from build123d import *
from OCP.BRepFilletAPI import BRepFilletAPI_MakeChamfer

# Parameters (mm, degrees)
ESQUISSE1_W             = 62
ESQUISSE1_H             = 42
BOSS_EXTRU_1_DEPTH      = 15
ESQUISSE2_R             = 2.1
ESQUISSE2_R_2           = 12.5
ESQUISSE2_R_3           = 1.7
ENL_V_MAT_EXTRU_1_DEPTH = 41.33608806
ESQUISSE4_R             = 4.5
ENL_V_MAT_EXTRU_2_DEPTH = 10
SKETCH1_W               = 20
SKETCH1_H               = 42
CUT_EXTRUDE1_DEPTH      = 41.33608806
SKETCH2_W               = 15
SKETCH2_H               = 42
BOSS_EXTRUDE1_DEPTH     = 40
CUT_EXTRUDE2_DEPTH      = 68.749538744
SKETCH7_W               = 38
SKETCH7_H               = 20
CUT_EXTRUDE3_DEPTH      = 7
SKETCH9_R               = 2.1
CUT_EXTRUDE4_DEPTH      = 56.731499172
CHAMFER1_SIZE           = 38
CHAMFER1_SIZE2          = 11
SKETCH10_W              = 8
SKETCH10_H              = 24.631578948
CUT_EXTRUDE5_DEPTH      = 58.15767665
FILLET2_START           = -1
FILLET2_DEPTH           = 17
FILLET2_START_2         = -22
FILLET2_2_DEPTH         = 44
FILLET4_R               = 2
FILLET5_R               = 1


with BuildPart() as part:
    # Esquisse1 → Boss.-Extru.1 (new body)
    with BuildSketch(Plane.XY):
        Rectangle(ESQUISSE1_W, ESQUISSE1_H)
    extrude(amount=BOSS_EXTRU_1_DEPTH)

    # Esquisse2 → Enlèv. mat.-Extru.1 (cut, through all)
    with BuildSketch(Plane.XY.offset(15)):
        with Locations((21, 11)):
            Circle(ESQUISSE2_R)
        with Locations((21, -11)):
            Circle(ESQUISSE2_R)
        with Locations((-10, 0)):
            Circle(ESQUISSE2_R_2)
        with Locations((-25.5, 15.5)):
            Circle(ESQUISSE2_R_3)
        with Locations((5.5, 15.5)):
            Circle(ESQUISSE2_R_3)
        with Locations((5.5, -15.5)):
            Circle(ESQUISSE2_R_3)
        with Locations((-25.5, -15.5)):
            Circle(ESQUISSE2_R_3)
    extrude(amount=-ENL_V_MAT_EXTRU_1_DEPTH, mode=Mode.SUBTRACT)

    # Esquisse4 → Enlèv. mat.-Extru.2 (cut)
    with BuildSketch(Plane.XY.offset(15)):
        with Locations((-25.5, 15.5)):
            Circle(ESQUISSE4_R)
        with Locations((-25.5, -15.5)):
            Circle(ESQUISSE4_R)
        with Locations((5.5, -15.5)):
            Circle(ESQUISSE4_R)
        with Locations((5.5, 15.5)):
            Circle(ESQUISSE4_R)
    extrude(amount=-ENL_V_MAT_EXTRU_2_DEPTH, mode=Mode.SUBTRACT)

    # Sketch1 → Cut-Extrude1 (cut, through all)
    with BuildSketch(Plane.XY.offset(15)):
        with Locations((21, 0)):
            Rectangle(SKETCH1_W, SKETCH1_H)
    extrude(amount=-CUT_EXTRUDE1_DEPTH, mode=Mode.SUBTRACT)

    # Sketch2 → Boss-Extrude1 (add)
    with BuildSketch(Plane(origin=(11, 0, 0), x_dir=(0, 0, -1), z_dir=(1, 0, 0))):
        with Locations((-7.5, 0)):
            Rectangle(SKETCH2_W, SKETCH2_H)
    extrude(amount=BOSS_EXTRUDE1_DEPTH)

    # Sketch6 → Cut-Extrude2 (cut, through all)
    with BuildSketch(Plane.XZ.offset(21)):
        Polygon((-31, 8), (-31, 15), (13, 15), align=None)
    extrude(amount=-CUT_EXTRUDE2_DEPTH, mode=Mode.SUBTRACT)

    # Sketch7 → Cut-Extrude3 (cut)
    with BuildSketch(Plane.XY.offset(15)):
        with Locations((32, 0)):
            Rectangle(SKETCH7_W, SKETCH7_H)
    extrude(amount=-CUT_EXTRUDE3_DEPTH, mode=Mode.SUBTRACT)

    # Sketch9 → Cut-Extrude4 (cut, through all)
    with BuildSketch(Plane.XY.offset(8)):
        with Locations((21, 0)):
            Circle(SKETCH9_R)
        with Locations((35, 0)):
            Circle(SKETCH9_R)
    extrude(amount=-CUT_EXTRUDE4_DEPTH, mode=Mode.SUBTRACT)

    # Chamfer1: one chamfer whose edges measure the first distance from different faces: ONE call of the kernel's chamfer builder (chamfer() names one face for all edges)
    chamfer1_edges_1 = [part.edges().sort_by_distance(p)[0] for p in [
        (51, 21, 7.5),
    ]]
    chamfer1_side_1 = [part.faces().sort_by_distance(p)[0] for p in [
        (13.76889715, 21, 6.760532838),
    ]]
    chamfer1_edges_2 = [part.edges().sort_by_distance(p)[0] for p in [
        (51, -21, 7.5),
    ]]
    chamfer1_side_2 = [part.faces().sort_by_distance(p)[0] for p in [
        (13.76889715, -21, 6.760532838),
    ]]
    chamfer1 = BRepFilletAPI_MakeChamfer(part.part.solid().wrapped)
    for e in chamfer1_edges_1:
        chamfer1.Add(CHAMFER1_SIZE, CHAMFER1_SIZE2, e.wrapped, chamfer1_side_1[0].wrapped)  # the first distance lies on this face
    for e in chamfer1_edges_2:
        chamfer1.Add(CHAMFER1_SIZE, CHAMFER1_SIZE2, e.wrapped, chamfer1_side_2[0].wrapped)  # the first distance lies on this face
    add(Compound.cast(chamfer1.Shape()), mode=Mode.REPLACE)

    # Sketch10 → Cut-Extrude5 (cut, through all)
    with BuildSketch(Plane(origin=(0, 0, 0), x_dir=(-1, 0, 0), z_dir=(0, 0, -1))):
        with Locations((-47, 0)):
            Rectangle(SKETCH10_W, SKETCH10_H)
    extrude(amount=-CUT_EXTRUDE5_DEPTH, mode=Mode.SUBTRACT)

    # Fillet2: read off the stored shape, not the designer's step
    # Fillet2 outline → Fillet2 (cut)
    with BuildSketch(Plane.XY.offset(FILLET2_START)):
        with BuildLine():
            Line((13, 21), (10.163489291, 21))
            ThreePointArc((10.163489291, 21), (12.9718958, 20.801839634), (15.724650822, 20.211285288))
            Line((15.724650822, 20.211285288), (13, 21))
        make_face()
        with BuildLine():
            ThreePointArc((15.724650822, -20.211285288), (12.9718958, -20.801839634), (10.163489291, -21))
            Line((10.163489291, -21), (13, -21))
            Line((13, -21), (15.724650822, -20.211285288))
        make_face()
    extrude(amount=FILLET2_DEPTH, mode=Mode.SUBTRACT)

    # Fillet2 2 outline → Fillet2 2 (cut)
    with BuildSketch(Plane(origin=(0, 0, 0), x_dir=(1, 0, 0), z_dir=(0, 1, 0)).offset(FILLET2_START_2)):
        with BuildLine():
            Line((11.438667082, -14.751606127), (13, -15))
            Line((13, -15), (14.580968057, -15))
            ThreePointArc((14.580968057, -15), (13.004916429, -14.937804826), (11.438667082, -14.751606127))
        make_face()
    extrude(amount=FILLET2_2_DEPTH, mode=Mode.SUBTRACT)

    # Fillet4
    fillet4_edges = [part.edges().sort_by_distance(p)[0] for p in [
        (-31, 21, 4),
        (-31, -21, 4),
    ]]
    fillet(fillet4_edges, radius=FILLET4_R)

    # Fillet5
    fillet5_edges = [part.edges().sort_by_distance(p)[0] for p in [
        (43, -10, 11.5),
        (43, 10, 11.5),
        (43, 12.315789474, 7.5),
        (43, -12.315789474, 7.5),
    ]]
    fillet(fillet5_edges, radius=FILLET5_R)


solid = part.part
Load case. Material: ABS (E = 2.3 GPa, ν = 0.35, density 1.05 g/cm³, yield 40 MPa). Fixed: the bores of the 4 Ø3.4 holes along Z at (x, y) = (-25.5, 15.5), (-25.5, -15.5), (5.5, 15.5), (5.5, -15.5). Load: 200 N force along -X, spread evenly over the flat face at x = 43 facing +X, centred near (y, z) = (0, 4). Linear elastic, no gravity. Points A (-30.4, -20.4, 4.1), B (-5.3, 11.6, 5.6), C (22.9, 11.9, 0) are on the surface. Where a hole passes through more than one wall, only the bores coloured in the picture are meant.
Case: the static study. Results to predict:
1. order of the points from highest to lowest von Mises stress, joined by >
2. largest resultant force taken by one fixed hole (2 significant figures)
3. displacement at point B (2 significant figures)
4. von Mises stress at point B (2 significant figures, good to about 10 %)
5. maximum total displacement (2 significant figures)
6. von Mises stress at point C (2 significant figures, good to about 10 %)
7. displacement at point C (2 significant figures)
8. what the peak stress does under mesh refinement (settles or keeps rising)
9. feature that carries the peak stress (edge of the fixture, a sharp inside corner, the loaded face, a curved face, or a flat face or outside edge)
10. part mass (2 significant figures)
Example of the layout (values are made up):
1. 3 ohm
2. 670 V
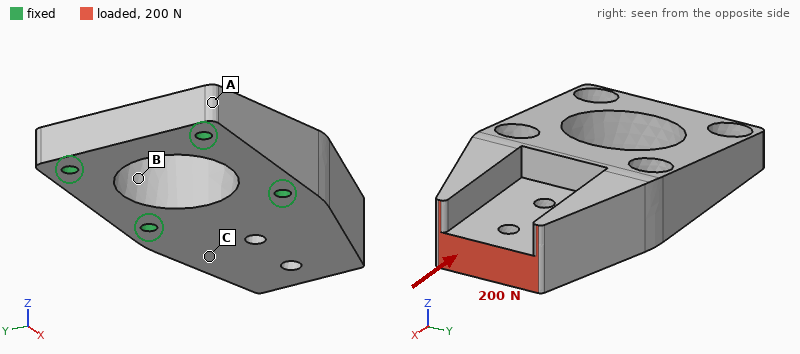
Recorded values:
1. C > B > A
2. 89 N
3. 3.5 µm
4. 0.54 MPa
5. 19 µm
6. 0.91 MPa
7. 8.5 µm
8. keeps rising
9. edge of the fixture
10. 26 g
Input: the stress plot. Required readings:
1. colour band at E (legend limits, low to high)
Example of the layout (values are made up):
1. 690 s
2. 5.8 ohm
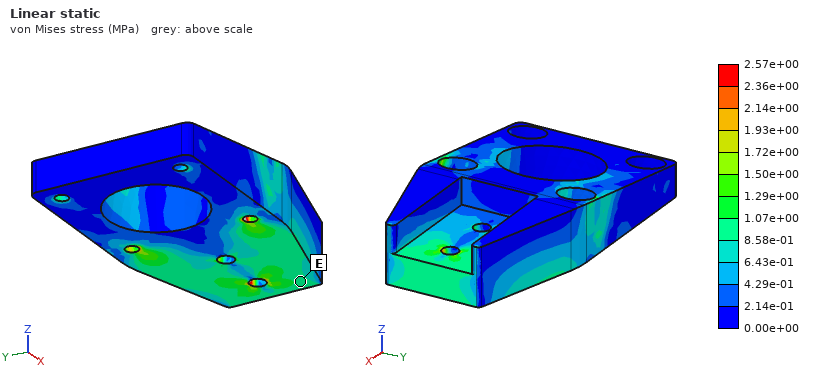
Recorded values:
1. 8.58e-01 to 1.07e+00 MPa
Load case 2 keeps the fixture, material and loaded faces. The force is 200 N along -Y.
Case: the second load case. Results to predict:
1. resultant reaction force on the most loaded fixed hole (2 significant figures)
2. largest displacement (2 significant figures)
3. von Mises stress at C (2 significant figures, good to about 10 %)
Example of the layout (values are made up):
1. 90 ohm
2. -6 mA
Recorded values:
1. 220 N
2. 85 µm
3. 1.9 MPa
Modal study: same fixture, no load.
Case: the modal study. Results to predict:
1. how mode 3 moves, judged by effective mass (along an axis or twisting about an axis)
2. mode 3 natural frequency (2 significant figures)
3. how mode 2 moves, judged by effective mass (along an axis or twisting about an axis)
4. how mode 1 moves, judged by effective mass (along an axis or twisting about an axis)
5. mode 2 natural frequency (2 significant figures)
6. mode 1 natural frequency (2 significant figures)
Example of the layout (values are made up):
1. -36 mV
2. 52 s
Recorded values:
1. along Y
2. 3900 Hz
3. twisting about X
4. along Z
5. 3500 Hz
6. 1500 Hz
